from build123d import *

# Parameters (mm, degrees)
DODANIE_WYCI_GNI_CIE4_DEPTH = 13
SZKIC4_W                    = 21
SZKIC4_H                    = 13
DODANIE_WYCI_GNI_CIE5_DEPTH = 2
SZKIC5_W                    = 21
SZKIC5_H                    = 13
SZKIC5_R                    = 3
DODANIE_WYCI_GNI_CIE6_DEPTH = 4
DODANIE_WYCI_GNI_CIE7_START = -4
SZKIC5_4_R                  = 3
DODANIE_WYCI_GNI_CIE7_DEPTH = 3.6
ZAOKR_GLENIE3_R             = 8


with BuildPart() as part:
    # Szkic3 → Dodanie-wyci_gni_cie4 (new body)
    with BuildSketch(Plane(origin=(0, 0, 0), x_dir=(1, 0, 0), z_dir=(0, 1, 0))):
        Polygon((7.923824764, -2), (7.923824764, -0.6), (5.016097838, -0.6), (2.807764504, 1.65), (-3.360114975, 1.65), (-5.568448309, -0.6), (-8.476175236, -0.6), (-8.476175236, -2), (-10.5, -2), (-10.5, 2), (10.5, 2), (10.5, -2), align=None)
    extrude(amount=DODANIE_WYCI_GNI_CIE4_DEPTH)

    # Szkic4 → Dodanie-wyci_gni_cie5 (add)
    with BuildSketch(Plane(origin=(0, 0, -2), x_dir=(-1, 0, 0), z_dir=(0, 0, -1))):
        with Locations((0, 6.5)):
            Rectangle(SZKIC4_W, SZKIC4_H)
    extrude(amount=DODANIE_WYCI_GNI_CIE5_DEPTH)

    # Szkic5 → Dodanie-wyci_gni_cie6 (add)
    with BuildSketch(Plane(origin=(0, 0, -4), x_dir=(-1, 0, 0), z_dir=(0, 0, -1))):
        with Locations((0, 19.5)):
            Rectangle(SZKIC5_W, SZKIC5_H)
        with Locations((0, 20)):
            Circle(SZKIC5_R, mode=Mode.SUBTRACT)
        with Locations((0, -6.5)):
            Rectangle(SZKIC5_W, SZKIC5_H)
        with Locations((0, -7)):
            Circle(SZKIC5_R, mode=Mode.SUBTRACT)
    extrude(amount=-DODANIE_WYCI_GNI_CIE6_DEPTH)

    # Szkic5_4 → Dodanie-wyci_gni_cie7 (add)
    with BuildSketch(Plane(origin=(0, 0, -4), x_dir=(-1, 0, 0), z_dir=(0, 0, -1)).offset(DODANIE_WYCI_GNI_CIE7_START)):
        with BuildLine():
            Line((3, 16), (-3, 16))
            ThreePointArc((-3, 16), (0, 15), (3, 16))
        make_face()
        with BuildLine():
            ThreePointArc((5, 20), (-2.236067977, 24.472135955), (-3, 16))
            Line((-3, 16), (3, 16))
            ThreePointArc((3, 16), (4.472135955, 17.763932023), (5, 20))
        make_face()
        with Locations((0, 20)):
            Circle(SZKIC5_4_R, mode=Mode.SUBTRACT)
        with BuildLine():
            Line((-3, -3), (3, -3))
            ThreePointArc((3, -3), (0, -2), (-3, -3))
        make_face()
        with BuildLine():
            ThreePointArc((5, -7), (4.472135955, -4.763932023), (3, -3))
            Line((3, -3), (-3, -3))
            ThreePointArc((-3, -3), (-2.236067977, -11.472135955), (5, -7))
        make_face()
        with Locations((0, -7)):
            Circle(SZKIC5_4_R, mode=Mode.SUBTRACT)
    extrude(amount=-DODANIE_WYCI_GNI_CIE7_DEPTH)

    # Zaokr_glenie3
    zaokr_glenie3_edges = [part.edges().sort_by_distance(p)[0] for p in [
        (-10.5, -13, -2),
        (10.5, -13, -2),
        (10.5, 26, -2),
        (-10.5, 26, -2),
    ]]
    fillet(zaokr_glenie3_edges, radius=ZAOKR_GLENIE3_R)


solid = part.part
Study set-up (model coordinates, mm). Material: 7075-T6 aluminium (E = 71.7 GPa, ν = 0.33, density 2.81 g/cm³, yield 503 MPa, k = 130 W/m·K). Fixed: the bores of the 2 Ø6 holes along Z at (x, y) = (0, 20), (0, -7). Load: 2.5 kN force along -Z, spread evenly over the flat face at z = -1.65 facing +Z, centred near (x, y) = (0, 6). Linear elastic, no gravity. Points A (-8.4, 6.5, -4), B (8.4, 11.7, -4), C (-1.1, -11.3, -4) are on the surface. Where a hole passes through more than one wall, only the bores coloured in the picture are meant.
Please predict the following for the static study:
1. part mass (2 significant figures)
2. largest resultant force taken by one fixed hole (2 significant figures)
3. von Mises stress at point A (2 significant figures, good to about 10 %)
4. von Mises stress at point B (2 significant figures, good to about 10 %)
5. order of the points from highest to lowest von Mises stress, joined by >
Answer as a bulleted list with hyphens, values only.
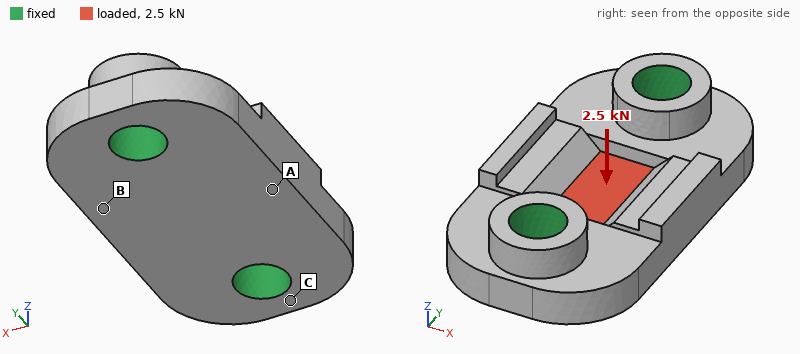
- 9.0 g
- 1.3 kN
- 46 MPa
- 32 MPa
- A > B > C
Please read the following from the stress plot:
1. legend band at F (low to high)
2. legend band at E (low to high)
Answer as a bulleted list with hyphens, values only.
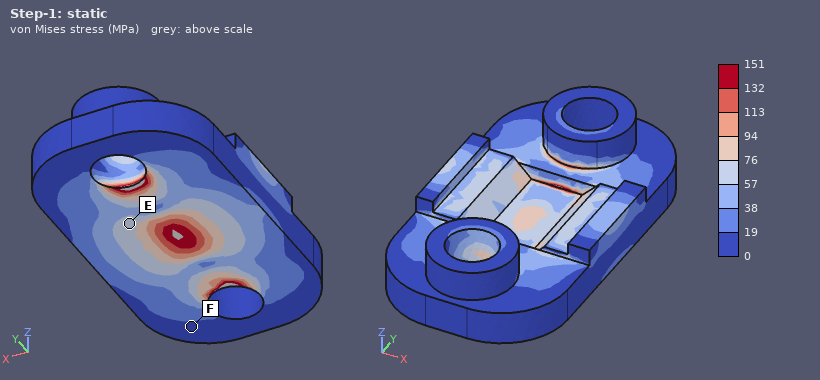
- 0 to 19 MPa
- 57 to 76 MPa
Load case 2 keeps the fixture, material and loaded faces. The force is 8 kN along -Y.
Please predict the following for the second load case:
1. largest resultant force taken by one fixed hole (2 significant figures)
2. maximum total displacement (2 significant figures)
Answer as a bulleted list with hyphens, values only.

- 4.0 kN
- 21 µm
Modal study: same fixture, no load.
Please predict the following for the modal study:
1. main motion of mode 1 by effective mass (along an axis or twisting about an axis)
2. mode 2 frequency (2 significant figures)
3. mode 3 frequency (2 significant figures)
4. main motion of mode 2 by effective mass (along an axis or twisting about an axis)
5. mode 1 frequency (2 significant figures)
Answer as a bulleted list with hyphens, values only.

- twisting about Y
- 27 kHz
- 49 kHz
- along Z
- 25 kHz
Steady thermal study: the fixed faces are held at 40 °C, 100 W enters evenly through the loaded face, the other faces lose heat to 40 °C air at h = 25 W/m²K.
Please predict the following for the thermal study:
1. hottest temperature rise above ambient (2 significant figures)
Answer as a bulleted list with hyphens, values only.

- 76 K
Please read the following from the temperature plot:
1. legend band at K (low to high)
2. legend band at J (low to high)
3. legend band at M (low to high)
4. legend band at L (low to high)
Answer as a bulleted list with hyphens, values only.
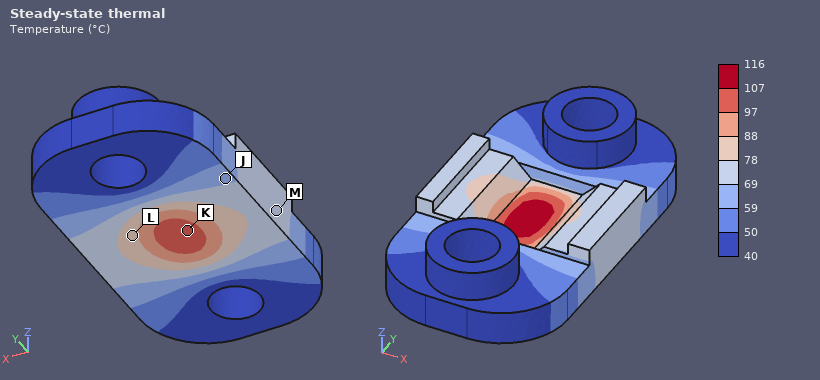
- 97 to 107 °C
- 59 to 69 °C
- 69 to 78 °C
- 78 to 88 °C
